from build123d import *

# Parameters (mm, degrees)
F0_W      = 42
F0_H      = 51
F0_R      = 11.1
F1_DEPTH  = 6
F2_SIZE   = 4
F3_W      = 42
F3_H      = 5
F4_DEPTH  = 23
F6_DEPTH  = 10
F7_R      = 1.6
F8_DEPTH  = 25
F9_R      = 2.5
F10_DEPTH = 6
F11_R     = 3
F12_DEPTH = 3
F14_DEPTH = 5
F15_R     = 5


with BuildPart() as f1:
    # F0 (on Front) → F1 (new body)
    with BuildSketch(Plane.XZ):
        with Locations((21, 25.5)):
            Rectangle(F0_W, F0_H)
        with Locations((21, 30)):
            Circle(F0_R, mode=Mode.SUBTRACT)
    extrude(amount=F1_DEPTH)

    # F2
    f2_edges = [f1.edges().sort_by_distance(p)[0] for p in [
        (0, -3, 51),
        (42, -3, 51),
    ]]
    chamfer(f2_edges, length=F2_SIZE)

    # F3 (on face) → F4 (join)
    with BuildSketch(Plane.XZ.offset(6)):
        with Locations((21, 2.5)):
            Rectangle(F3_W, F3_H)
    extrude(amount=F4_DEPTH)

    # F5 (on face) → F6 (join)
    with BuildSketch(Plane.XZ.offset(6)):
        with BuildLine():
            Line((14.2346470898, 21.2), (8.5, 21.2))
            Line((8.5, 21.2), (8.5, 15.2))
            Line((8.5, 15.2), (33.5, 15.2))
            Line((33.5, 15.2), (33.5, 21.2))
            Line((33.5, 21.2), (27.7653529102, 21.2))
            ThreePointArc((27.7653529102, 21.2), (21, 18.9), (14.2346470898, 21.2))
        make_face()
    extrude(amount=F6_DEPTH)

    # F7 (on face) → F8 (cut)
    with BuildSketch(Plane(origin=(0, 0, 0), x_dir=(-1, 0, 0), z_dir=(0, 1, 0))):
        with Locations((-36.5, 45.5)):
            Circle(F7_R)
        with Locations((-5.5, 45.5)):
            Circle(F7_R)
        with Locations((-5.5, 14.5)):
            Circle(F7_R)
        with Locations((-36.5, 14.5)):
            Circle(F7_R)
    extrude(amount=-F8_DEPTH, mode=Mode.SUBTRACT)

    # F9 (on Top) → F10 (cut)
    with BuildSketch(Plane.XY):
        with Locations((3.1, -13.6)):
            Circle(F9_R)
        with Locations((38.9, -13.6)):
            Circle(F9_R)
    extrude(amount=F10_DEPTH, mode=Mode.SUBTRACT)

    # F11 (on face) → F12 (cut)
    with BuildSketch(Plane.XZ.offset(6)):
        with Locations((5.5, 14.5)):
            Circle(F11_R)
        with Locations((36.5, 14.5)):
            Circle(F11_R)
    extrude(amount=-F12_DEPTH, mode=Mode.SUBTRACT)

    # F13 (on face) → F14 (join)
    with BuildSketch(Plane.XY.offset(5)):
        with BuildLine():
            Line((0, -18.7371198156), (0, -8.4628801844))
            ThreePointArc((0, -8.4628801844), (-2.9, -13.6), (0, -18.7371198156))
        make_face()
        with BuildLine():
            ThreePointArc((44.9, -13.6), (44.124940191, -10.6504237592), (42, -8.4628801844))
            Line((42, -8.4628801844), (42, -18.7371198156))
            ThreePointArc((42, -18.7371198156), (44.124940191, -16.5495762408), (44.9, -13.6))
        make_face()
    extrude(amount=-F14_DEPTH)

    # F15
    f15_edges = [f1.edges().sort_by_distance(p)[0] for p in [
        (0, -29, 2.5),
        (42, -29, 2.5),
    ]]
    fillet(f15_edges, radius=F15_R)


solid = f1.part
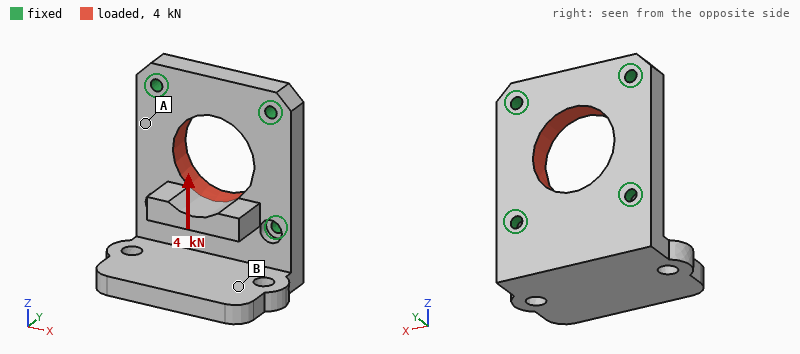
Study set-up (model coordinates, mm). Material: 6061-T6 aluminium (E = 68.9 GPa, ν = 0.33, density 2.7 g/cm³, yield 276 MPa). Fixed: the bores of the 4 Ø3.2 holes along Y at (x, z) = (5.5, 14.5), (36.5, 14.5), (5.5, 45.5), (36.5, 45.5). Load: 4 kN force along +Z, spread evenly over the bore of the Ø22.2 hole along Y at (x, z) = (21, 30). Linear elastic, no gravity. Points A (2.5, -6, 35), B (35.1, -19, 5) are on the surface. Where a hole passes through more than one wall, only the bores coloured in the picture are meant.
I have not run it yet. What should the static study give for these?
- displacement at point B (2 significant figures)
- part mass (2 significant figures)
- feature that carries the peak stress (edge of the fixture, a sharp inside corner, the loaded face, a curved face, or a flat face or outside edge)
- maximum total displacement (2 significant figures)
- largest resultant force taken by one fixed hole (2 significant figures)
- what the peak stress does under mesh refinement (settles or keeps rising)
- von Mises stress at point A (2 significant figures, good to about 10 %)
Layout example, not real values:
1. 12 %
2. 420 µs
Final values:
1. 9.2 µm
2. 44 g
3. edge of the fixture
4. 14 µm
5. 1.1 kN
6. keeps rising
7. 9.7 MPa
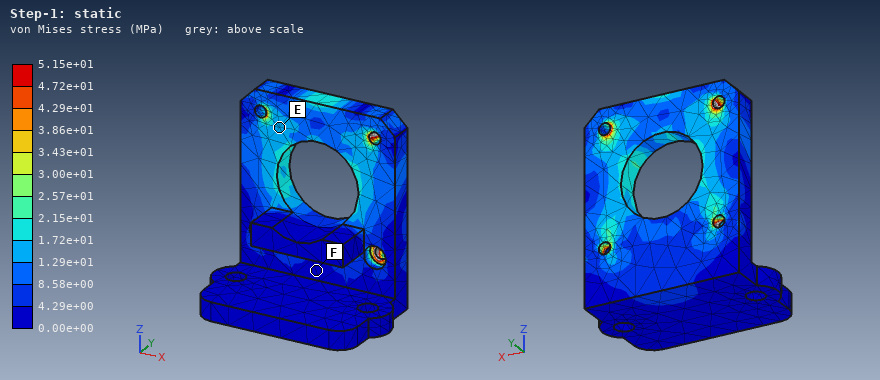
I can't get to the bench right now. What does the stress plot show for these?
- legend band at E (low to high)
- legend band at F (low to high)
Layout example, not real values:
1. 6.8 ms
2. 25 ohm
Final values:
1. 1.29e+01 to 1.72e+01 MPa
2. 0.00e+00 to 4.29e+00 MPa
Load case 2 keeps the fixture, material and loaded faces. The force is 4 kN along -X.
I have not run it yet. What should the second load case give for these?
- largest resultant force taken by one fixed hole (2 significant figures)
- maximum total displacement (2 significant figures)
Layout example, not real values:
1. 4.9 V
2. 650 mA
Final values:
1. 1.0 kN
2. 7.0 µm
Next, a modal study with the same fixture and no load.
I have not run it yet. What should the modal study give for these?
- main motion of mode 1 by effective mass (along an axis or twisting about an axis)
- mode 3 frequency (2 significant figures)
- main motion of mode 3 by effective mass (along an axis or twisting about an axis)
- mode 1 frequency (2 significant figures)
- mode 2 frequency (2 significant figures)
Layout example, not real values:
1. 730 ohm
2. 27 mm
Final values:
1. along Z
2. 9900 Hz
3. along Y
4. 3400 Hz
5. 6900 Hz
